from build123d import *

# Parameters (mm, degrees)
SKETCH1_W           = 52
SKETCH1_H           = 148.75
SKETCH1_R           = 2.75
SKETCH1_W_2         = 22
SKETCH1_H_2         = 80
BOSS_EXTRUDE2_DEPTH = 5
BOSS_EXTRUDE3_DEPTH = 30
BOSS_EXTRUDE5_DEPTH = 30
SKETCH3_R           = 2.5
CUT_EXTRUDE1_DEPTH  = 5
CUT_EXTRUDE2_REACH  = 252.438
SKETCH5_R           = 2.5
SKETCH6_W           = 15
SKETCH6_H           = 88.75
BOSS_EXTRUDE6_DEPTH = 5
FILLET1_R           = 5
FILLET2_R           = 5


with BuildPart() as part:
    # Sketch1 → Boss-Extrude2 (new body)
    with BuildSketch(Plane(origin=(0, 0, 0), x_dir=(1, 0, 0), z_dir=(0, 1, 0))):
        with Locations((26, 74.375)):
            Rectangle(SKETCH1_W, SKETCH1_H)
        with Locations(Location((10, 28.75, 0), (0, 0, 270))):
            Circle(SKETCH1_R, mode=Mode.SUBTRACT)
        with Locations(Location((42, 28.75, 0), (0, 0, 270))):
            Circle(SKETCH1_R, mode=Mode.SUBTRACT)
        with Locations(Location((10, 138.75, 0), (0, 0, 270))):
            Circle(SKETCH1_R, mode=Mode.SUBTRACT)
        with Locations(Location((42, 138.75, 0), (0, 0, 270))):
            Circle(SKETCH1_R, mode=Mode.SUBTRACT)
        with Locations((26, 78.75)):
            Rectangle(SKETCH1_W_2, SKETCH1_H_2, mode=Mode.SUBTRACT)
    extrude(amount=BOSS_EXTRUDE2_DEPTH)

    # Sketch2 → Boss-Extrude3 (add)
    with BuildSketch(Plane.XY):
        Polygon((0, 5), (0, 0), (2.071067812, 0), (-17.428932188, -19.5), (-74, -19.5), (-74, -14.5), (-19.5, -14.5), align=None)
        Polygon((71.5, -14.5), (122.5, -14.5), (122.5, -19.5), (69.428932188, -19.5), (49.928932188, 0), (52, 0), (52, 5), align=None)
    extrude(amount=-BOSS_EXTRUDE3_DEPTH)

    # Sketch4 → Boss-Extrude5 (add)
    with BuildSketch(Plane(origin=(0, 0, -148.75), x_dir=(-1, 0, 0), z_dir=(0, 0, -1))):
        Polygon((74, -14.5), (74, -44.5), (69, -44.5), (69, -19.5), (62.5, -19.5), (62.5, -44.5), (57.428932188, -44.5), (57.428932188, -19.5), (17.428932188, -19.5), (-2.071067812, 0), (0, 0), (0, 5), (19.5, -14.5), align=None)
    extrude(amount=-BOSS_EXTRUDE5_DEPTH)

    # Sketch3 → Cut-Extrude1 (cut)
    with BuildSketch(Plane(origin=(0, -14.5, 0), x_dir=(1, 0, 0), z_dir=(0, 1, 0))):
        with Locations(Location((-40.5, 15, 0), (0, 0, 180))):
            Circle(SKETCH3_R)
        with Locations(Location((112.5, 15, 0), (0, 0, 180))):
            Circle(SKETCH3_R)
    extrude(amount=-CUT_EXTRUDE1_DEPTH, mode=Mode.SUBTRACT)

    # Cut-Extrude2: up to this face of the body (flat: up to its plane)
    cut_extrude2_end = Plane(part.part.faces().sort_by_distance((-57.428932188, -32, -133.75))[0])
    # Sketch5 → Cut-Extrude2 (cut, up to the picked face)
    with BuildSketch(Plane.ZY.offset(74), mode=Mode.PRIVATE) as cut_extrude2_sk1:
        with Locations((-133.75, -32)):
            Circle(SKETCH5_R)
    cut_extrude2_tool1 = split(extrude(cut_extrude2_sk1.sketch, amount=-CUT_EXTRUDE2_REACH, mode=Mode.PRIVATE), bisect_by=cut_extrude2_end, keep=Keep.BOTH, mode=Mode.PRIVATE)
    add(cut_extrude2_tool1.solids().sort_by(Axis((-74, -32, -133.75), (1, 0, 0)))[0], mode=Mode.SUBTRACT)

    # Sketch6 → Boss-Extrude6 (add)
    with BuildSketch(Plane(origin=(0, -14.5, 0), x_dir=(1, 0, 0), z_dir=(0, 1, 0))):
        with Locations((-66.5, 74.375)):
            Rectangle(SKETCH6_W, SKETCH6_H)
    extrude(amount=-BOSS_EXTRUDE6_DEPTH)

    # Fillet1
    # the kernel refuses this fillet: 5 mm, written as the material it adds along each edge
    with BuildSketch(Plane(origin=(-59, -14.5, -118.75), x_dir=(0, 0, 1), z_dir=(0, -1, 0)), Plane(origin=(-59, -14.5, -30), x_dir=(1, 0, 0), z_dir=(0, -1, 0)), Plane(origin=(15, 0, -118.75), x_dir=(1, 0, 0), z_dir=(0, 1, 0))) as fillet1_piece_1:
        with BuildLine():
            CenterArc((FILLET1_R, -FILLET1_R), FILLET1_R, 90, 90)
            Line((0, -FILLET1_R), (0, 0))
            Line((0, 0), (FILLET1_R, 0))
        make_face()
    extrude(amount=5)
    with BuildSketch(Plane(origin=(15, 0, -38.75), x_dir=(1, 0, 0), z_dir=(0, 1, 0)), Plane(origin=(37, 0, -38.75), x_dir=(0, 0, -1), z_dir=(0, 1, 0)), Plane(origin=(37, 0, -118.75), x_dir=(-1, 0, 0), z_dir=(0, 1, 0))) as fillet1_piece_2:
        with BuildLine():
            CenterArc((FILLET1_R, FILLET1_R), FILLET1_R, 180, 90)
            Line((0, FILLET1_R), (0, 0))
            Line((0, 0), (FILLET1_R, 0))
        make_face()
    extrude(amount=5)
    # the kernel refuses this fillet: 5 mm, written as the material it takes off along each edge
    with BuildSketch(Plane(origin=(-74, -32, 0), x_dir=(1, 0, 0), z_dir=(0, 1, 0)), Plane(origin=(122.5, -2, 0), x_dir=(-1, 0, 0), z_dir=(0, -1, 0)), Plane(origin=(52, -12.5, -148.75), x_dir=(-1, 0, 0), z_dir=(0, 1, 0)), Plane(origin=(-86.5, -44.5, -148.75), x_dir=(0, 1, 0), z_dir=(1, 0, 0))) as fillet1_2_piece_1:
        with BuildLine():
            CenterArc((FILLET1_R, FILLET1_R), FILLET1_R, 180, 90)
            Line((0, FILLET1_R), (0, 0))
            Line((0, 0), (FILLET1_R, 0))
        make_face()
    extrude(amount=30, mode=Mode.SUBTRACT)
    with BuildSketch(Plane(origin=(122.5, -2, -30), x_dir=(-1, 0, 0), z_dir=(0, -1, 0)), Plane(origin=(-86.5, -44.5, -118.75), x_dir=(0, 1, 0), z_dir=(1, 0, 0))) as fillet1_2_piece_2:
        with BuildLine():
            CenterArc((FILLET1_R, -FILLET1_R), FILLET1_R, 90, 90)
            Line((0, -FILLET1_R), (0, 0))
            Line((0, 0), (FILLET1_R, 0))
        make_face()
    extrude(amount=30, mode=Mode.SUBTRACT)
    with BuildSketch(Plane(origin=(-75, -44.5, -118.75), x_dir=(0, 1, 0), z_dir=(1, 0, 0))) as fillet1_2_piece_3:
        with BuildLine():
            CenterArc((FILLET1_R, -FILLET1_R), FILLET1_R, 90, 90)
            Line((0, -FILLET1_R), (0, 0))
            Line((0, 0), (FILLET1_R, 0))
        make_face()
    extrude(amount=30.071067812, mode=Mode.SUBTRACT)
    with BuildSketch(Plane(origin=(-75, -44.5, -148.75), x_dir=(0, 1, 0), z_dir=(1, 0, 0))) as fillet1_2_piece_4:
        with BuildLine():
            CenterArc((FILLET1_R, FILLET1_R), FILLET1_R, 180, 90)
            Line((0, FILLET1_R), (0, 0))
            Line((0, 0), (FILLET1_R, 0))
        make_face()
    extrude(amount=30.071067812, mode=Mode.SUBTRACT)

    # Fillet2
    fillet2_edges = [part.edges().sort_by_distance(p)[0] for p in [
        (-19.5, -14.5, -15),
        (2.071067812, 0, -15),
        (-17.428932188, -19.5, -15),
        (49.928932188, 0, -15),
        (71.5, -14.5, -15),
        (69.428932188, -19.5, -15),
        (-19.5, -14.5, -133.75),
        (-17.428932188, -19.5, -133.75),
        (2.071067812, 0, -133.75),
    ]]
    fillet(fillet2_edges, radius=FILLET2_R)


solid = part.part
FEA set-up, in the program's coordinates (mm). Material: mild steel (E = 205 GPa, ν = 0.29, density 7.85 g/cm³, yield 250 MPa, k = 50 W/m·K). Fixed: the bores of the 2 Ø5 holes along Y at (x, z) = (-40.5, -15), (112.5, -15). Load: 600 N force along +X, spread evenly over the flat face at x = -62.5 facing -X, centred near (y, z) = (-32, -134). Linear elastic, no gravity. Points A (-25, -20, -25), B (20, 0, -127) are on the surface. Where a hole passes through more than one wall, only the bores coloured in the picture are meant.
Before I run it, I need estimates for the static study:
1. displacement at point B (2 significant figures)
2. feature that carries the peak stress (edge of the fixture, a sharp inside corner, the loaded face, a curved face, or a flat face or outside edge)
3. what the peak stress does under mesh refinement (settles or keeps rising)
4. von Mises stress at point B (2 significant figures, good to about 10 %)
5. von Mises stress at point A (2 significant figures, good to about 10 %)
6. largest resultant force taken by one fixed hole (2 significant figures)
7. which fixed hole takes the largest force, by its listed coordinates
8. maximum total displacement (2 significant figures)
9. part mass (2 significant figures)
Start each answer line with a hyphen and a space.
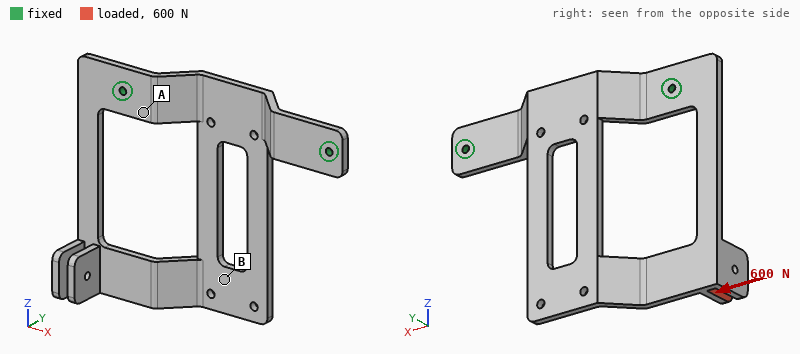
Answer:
- 0.16 mm
- edge of the fixture
- keeps rising
- 44 MPa
- 17 MPa
- 670 N
- (-40.5, -15)
- 1.0 mm
- 630 g
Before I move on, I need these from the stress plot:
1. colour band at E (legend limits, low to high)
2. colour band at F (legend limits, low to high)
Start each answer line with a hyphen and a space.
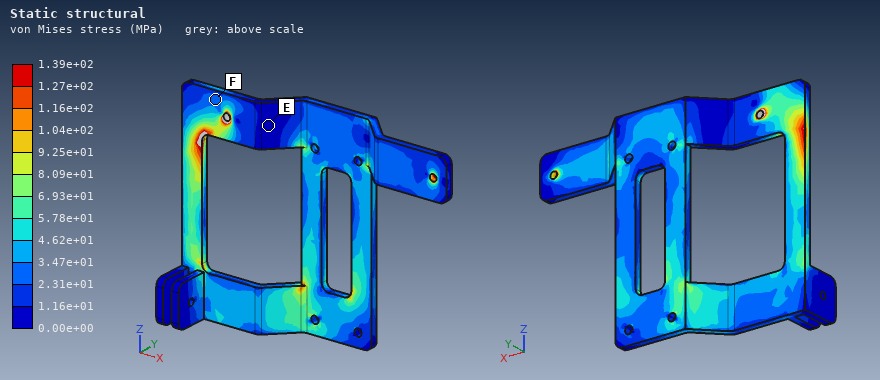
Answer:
- 0.00e+00 to 1.16e+01 MPa
- 2.31e+01 to 3.47e+01 MPa
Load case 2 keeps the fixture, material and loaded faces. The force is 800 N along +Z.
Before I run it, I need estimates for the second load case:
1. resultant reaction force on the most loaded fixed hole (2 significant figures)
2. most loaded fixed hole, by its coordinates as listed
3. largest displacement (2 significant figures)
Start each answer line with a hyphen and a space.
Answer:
- 810 N
- (-40.5, -15)
- 1.1 mm
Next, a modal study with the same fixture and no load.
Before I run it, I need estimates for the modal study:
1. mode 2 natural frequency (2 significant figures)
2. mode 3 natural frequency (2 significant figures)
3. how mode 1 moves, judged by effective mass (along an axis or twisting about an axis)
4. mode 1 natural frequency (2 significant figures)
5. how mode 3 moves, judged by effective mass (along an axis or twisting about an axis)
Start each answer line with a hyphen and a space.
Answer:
- 330 Hz
- 650 Hz
- along Y
- 140 Hz
- along X
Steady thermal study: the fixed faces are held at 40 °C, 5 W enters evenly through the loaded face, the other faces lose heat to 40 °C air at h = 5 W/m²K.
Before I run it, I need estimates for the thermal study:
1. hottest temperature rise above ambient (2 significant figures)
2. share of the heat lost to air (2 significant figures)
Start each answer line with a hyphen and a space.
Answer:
- 51 K
- 59 %
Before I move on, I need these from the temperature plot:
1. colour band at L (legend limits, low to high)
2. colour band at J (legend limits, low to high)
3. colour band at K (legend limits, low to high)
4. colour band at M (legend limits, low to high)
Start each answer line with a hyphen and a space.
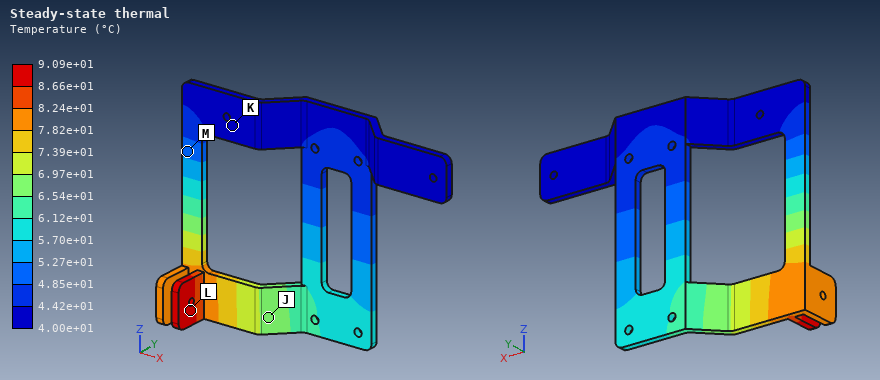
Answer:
- 8.66e+01 to 9.09e+01 °C
- 6.54e+01 to 6.97e+01 °C
- 4.00e+01 to 4.42e+01 °C
- 4.85e+01 to 5.27e+01 °C
